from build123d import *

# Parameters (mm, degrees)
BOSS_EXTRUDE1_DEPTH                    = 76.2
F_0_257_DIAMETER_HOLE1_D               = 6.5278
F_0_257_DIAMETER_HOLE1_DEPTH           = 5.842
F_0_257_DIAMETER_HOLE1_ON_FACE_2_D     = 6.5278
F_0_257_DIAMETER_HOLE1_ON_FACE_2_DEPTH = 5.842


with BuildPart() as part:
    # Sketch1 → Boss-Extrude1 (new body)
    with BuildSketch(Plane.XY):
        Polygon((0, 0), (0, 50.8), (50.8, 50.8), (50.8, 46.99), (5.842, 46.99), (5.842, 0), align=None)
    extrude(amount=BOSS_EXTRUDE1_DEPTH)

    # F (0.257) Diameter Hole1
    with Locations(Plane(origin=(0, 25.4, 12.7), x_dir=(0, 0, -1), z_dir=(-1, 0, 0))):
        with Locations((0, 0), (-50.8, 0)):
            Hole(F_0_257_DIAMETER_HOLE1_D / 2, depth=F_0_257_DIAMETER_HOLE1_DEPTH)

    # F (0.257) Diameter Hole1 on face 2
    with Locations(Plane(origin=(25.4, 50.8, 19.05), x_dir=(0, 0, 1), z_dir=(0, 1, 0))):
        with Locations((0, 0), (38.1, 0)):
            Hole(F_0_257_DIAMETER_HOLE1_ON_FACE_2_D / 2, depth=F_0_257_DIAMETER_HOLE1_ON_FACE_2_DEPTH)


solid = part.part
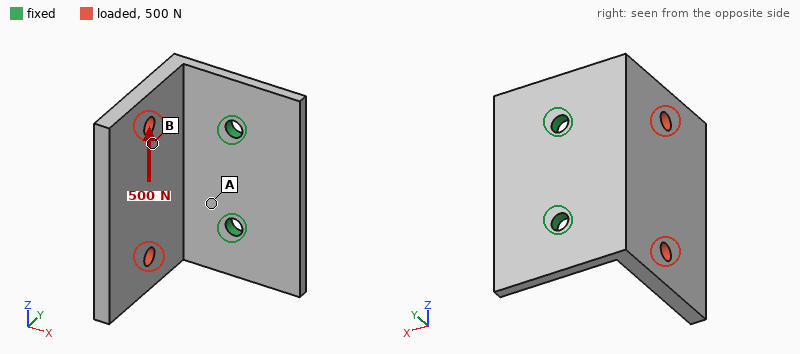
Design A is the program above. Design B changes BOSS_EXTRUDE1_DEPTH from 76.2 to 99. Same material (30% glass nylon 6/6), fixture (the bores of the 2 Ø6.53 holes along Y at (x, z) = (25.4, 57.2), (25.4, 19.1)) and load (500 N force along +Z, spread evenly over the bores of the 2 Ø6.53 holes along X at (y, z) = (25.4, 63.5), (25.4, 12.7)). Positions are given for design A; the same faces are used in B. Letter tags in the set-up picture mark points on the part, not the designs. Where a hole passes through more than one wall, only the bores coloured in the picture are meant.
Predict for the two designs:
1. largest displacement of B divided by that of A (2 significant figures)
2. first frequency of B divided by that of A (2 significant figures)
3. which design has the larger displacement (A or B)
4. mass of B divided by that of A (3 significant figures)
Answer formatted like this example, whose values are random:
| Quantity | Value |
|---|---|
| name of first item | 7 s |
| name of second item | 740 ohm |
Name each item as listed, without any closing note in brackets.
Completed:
| Quantity | Value |
|---|---|
| largest displacement of B divided by that of A | 1.2 |
| first frequency of B divided by that of A | 0.93 |
| which design has the larger displacement | B |
| mass of B divided by that of A | 1.30 |
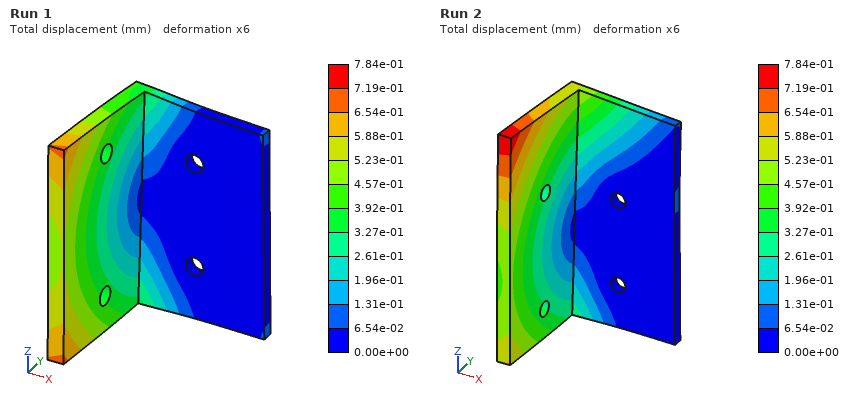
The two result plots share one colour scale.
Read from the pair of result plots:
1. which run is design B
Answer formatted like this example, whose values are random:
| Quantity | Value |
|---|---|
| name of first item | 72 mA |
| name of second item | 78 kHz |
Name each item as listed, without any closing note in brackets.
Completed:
| Quantity | Value |
|---|---|
| which run is design B | Run 2 |
